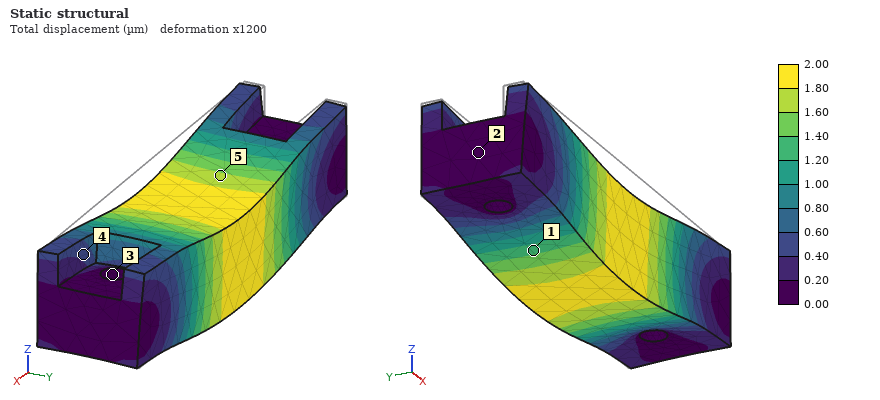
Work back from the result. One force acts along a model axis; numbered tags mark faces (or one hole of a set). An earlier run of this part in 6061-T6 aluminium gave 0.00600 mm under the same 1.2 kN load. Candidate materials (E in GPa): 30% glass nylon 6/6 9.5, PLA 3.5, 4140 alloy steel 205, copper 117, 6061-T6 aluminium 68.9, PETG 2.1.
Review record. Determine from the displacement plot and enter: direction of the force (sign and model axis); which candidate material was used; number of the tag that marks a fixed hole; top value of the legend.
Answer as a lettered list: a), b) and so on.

a) -Z
b) 4140 alloy steel
c) 3
d) 2.00 µm
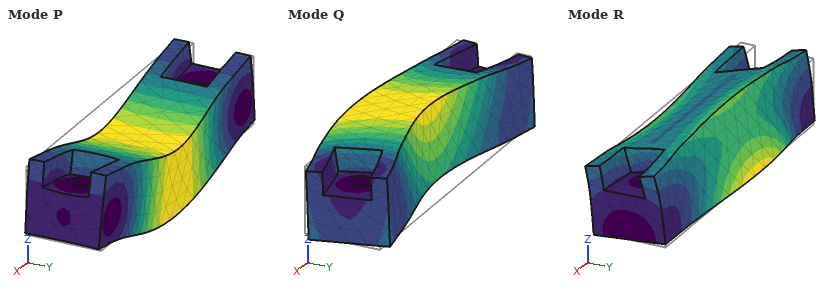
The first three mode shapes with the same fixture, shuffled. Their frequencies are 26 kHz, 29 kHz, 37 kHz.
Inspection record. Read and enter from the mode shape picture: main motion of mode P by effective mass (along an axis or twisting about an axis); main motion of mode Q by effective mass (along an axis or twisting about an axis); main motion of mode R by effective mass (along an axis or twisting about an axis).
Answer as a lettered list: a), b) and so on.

a) along Z
b) along Y
c) twisting about X
